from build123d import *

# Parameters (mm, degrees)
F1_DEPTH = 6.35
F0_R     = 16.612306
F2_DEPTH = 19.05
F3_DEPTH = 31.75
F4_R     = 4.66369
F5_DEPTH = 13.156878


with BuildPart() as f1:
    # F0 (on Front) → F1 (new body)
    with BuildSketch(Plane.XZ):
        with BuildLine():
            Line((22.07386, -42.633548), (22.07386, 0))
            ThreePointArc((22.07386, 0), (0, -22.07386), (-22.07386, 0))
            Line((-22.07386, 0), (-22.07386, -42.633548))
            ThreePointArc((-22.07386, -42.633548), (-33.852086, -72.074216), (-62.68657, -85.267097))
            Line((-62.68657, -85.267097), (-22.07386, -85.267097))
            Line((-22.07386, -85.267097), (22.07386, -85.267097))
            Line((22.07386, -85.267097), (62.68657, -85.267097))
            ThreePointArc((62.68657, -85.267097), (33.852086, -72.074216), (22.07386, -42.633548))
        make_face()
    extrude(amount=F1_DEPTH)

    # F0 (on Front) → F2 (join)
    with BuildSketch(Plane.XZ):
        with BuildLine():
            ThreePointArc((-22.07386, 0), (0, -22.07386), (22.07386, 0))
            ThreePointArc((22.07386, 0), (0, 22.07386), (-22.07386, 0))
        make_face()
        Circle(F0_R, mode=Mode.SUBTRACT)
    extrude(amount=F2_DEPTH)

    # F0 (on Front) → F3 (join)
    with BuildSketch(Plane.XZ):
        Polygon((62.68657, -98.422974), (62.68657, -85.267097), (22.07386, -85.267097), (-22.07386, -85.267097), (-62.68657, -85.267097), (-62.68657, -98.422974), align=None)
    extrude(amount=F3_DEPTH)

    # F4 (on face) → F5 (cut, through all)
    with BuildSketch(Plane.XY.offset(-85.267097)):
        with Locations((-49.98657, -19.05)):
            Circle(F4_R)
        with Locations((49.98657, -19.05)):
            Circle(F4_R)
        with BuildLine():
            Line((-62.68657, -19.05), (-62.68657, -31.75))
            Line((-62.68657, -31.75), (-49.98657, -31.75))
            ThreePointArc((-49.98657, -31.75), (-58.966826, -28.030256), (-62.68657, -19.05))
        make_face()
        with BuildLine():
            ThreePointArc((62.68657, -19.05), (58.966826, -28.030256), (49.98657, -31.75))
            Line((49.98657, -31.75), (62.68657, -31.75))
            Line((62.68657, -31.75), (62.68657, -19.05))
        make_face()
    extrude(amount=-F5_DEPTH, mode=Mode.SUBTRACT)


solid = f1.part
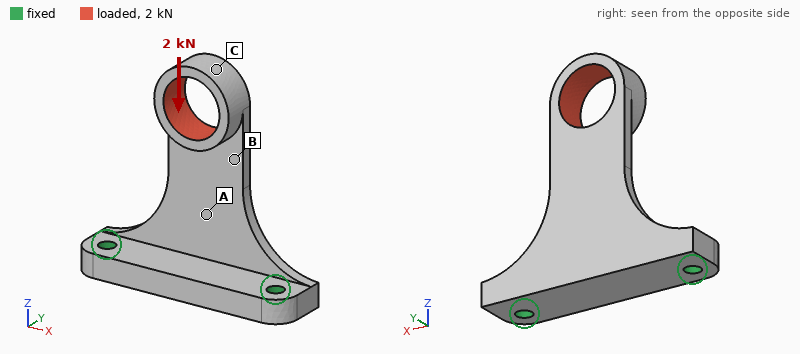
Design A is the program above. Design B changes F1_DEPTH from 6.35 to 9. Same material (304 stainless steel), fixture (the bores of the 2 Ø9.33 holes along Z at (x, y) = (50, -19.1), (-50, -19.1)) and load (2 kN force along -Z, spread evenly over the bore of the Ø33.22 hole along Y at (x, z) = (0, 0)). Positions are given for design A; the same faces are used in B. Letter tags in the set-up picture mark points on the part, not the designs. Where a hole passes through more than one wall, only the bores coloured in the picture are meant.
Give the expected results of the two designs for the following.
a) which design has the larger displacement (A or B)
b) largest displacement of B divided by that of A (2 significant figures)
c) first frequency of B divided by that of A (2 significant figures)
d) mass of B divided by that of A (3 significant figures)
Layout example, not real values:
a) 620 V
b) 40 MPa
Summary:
a) A
b) 0.28
c) 1.5
d) 1.12
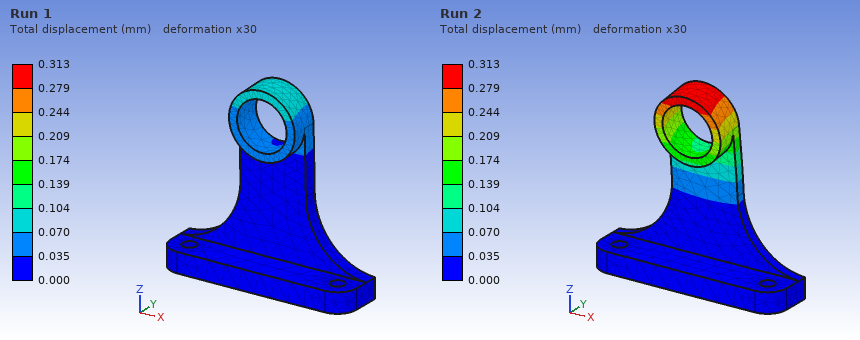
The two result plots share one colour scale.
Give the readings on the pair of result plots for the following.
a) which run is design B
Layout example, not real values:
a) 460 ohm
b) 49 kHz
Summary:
a) Run 1
